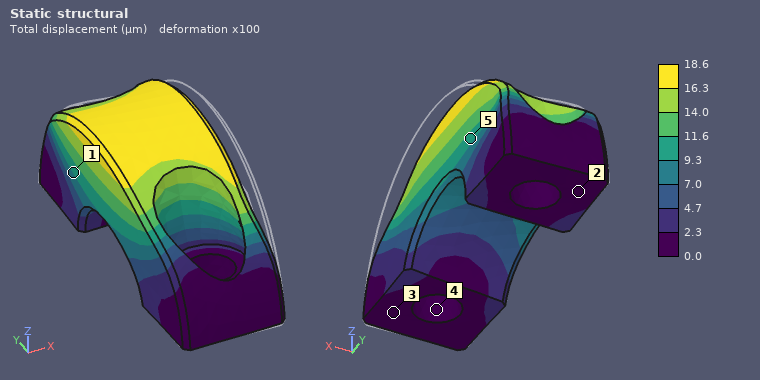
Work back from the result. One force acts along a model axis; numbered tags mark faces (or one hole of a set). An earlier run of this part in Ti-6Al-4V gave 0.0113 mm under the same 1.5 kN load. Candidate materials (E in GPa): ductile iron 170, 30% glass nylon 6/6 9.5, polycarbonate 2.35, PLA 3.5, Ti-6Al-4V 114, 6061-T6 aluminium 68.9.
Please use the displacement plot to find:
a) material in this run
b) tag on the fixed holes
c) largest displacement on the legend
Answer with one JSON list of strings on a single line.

["6061-T6 aluminium", "4", "18.6 µm"]
